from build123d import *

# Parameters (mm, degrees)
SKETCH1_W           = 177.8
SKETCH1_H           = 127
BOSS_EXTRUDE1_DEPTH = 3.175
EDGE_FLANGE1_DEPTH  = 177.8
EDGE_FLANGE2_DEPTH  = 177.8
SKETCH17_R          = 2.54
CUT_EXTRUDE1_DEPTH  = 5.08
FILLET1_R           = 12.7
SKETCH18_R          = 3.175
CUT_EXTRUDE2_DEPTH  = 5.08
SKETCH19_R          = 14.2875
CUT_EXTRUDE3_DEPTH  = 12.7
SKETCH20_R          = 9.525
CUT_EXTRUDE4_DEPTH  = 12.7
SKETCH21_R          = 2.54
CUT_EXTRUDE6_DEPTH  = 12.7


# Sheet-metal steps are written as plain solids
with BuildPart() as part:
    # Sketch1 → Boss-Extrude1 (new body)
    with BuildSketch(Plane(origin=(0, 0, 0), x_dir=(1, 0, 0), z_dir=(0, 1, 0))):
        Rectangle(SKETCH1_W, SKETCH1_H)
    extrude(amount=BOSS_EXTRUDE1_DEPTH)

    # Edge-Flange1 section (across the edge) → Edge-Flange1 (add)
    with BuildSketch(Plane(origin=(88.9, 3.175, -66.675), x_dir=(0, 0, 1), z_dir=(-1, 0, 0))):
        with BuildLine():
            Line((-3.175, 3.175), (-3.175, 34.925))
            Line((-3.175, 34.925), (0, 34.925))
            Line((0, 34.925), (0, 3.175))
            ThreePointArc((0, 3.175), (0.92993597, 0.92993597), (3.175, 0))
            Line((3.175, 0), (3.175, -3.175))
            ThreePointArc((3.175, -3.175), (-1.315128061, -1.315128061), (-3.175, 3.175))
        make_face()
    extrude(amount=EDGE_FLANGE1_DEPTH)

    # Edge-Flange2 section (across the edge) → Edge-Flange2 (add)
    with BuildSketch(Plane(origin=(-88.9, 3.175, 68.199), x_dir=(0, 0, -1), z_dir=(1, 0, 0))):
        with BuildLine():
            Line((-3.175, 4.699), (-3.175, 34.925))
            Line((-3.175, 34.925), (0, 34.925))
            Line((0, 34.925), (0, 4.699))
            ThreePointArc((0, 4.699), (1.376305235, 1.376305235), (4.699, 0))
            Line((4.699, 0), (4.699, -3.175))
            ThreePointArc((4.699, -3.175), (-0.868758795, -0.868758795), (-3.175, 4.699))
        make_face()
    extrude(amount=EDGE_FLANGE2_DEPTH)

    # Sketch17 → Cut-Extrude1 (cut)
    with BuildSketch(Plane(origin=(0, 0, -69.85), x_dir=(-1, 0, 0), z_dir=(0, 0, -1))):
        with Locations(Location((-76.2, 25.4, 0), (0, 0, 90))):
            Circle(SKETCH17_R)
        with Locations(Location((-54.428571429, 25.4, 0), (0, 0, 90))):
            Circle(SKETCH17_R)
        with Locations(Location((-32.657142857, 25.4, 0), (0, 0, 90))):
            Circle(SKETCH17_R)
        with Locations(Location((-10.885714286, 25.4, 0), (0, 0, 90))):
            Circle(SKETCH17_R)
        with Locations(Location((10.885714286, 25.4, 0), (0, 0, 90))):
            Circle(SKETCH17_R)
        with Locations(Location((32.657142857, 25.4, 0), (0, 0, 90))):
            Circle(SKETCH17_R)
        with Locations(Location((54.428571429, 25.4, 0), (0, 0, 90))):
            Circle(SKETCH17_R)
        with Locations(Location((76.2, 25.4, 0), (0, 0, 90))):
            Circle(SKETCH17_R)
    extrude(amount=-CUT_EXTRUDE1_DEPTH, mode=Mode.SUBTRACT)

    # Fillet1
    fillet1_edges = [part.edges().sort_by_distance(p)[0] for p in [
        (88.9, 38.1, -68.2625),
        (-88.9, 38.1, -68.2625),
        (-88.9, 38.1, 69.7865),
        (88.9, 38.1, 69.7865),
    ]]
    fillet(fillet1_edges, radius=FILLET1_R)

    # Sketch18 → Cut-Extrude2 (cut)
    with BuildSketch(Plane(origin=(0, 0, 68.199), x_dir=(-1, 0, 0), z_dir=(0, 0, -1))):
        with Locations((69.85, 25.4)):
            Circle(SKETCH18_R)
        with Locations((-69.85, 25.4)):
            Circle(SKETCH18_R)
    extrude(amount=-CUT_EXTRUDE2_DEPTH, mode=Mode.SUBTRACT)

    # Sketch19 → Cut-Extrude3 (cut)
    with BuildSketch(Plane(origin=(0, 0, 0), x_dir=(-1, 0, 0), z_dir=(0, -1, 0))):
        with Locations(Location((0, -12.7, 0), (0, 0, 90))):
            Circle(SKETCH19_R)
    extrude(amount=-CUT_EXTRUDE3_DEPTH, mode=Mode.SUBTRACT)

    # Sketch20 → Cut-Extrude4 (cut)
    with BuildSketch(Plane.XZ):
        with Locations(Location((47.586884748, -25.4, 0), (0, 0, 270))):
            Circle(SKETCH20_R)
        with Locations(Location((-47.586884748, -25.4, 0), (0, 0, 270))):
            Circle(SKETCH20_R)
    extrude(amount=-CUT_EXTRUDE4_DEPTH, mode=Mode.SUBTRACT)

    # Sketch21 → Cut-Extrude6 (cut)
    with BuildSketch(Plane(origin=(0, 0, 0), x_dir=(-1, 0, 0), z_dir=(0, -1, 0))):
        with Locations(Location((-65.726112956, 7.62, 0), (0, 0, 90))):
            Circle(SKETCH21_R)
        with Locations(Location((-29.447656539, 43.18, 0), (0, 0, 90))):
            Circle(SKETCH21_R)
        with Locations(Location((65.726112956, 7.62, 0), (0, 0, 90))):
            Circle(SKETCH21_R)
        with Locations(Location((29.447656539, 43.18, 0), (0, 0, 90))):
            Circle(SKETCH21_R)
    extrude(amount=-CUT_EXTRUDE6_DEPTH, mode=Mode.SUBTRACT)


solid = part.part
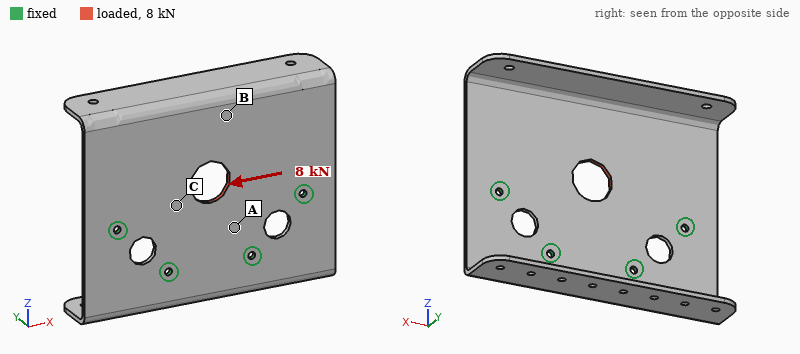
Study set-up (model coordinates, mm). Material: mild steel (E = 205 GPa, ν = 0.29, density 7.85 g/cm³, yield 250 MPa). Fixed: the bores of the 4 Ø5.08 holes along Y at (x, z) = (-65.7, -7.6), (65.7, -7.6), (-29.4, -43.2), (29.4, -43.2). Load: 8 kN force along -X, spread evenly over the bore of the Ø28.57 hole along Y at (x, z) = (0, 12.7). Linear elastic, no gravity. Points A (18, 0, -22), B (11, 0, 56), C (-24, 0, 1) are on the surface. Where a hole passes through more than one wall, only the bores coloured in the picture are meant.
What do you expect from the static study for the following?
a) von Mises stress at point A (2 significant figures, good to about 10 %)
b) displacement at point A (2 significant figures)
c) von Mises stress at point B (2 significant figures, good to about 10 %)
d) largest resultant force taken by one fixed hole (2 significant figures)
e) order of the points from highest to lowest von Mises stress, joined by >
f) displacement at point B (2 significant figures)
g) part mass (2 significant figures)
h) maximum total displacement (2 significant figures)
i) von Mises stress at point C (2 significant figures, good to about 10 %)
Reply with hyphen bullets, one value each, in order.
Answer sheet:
- 18 MPa
- 3.3 µm
- 6.5 MPa
- 3.3 kN
- C > A > B
- 10 µm
- 870 g
- 13 µm
- 27 MPa
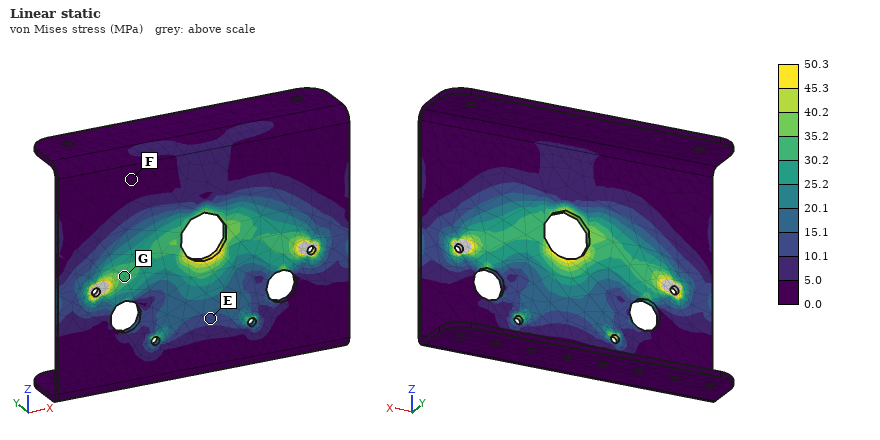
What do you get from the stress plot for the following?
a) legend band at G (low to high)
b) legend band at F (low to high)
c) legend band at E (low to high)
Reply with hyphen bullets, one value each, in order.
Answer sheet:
- 30.2 to 35.2 MPa
- 0.0 to 5.0 MPa
- 10.1 to 15.1 MPa
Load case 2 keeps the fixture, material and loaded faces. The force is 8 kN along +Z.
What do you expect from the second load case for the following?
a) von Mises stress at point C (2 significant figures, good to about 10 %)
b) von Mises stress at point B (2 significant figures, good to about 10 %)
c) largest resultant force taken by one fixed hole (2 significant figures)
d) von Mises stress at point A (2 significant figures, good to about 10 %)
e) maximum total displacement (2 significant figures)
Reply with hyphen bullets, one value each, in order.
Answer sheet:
- 22 MPa
- 14 MPa
- 2.5 kN
- 24 MPa
- 11 µm
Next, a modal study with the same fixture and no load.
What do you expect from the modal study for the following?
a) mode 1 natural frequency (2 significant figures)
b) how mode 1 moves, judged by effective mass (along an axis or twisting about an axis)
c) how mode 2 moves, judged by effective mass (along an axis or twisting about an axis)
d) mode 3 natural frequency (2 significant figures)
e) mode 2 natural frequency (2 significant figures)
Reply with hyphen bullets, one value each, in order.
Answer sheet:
- 220 Hz
- along Y
- twisting about Z
- 810 Hz
- 400 Hz
